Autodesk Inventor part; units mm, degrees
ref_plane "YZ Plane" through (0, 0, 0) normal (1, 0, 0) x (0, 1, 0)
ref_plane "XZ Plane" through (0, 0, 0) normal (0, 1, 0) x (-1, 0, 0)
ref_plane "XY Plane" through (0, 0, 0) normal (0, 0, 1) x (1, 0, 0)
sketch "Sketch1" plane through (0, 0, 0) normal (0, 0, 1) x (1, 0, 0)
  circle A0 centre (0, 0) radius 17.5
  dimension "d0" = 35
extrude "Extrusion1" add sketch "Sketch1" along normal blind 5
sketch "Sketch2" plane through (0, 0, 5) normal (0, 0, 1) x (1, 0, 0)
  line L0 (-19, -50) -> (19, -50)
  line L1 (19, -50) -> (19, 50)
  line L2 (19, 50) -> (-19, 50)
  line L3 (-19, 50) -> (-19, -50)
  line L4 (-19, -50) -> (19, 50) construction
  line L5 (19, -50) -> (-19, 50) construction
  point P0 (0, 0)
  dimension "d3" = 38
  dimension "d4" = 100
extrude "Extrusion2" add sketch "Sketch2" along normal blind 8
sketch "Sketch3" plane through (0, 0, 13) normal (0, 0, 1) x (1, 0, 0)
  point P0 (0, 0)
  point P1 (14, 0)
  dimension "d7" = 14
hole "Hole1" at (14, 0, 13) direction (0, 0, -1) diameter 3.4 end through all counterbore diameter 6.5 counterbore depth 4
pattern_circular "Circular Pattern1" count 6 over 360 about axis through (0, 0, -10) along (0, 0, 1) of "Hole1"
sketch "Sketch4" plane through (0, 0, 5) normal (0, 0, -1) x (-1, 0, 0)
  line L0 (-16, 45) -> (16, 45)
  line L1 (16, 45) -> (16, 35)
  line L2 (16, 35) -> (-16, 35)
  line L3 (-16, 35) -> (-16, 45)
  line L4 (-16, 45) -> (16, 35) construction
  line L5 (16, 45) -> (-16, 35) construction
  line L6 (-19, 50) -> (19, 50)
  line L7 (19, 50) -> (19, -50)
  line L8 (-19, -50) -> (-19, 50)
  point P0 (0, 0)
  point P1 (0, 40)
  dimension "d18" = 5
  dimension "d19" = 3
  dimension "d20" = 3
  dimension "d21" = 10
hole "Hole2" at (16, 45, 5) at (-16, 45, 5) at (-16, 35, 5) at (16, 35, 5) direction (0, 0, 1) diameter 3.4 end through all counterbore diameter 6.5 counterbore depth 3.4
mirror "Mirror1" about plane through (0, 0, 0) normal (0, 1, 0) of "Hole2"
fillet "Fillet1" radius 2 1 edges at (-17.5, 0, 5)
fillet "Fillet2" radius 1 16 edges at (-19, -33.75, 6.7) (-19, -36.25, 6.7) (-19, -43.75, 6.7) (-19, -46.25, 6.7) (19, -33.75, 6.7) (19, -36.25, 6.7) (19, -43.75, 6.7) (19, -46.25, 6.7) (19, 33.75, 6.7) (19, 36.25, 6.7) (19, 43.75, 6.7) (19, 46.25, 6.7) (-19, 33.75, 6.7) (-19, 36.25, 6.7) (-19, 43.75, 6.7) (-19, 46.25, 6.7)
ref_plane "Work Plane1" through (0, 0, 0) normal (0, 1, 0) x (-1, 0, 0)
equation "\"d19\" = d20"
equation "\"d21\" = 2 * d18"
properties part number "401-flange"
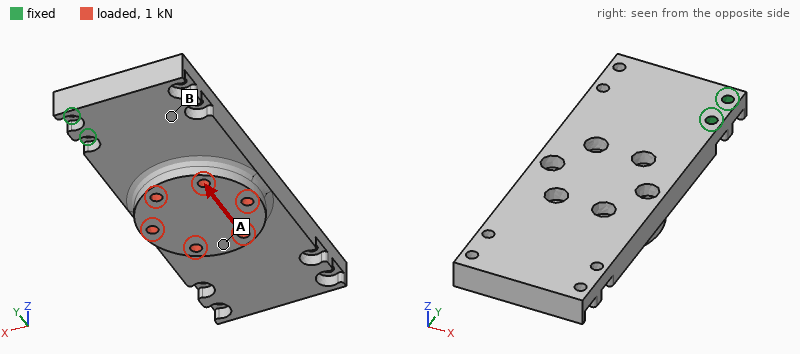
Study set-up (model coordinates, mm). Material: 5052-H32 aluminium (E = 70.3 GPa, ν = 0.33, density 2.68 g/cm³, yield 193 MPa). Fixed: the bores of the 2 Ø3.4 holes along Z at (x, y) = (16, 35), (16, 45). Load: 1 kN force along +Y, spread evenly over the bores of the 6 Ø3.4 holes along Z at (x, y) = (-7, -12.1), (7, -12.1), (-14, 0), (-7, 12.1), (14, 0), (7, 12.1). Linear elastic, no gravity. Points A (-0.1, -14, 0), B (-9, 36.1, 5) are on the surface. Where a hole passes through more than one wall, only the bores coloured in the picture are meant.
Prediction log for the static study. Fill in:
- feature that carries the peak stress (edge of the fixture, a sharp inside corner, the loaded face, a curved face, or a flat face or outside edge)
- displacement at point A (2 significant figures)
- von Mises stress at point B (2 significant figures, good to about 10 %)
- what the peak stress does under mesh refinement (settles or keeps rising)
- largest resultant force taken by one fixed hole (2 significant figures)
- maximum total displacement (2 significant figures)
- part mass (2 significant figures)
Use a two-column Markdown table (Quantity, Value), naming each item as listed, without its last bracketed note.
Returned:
| Quantity | Value |
|---|---|
| feature that carries the peak stress | edge of the fixture |
| displacement at point A | 0.081 mm |
| von Mises stress at point B | 13 MPa |
| what the peak stress does under mesh refinement | keeps rising |
| largest resultant force taken by one fixed hole | 1.4 kN |
| maximum total displacement | 0.15 mm |
| part mass | 88 g |
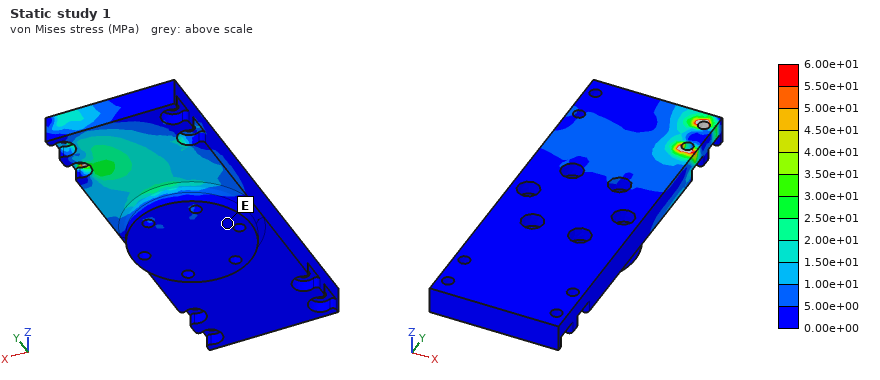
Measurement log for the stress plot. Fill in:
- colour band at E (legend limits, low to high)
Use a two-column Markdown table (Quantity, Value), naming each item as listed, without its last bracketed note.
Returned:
| Quantity | Value |
|---|---|
| colour band at E | 0.00e+00 to 5.00e+00 MPa |
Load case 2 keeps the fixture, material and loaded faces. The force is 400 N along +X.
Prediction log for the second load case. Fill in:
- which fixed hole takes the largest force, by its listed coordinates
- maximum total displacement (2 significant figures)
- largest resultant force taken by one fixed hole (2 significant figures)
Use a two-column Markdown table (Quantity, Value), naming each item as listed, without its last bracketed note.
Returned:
| Quantity | Value |
|---|---|
| which fixed hole takes the largest force, by its listed coordinates | (16, 35) |
| maximum total displacement | 0.10 mm |
| largest resultant force taken by one fixed hole | 1.4 kN |
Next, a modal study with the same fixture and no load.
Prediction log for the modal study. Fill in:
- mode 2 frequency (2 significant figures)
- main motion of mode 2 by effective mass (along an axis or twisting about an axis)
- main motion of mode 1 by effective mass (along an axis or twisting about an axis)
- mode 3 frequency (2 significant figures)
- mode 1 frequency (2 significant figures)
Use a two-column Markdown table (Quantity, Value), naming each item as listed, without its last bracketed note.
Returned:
| Quantity | Value |
|---|---|
| mode 2 frequency | 1500 Hz |
| main motion of mode 2 by effective mass | along X |
| main motion of mode 1 by effective mass | along Z |
| mode 3 frequency | 2200 Hz |
| mode 1 frequency | 640 Hz |
